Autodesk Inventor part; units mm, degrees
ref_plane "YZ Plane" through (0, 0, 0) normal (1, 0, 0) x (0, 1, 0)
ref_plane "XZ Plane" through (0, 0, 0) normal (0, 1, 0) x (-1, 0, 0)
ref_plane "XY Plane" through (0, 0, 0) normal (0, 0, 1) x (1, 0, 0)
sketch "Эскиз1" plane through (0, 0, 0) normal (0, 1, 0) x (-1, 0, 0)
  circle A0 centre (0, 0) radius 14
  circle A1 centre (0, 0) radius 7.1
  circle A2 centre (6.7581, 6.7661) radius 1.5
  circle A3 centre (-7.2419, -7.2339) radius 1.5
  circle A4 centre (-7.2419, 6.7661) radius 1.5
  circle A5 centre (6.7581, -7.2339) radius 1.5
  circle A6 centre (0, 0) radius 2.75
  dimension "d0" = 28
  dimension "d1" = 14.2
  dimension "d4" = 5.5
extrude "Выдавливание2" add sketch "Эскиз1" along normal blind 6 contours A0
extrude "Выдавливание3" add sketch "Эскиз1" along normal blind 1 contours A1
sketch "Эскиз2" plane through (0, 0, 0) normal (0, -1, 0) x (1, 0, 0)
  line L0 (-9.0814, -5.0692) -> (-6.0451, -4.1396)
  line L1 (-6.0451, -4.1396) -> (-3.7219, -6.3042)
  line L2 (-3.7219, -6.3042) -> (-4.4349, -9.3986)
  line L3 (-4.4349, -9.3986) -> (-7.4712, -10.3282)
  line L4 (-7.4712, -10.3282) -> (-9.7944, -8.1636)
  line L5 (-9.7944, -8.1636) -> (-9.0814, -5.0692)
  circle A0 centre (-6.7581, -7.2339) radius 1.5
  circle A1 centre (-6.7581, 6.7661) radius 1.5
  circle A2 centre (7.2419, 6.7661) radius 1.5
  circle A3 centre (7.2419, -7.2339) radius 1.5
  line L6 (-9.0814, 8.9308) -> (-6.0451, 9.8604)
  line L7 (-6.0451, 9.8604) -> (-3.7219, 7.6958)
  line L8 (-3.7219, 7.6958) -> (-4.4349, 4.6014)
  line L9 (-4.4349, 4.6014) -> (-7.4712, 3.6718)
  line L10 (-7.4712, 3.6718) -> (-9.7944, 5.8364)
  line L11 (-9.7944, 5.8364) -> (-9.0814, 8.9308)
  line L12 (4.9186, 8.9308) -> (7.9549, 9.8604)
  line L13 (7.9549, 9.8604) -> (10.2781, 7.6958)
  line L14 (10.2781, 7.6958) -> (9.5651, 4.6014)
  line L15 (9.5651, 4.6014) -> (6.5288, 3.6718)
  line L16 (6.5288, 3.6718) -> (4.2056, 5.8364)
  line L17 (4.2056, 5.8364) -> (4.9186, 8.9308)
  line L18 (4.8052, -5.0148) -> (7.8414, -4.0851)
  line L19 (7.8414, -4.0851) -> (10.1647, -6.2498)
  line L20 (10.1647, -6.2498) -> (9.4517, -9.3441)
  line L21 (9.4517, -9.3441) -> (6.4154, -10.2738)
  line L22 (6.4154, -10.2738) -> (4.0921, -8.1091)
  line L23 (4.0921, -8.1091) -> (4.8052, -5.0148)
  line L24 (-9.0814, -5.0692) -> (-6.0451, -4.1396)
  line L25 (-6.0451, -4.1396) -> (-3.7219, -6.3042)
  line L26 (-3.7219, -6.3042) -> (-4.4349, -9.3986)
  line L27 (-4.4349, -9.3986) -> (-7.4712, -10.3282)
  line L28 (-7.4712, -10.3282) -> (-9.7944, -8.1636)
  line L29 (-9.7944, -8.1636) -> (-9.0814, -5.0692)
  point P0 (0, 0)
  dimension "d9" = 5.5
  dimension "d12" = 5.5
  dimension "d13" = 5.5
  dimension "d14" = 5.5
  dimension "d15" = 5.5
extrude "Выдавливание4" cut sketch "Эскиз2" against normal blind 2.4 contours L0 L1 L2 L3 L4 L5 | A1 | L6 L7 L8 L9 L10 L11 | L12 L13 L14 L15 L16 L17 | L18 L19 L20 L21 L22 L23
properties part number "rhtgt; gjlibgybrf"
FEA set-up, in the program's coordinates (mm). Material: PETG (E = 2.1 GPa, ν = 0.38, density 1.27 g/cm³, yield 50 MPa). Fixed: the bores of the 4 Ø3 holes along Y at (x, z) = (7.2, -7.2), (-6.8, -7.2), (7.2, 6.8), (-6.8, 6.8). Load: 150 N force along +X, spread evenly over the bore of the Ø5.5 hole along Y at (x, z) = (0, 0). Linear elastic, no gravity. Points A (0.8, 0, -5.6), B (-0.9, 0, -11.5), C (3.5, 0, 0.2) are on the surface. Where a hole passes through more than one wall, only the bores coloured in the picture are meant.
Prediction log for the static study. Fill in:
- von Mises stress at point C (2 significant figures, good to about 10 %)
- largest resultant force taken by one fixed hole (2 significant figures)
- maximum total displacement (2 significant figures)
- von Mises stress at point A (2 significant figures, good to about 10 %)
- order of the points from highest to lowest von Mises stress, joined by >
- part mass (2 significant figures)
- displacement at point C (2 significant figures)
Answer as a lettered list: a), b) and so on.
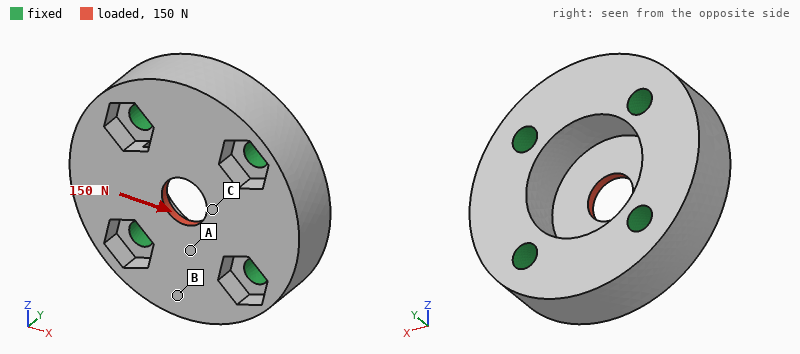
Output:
a) 9.5 MPa
b) 40 N
c) 43 µm
d) 4.5 MPa
e) C > A > B
f) 3.2 g
g) 39 µm
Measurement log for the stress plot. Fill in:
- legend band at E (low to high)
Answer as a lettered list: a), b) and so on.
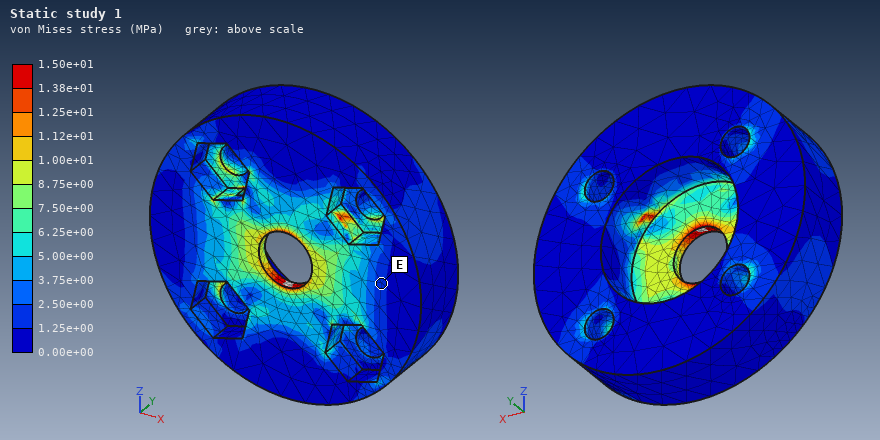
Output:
a) 1.25e+00 to 2.50e+00 MPa
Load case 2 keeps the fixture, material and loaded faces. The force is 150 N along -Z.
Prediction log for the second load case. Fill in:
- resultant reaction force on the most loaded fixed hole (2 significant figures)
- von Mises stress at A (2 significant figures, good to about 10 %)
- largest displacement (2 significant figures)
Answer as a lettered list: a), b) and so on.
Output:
a) 40 N
b) 6.7 MPa
c) 43 µm
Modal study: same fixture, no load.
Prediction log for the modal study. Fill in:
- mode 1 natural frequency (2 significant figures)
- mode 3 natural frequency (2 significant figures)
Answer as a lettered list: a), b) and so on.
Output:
a) 11 kHz
b) 12 kHz
